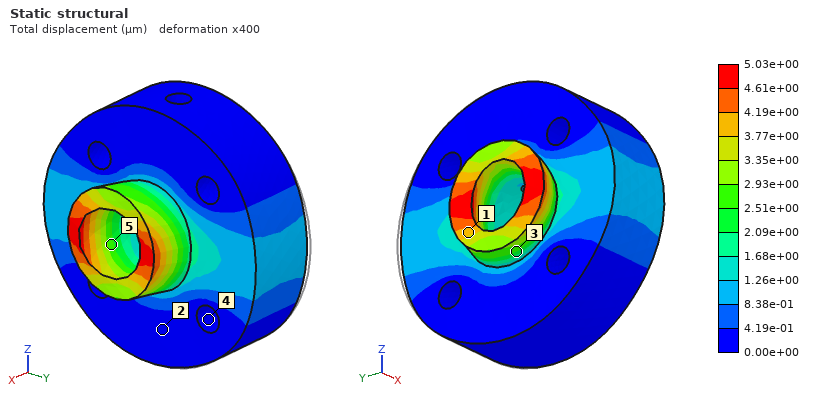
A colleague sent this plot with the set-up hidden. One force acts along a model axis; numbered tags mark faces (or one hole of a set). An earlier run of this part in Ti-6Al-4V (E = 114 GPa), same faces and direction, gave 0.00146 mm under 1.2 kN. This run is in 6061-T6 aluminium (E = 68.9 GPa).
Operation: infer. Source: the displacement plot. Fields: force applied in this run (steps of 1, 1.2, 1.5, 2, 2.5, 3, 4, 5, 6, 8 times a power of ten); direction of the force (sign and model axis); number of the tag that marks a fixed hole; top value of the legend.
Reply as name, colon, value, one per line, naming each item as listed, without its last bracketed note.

force applied in this run: 2.5 kN
direction of the force: -Y
number of the tag that marks a fixed hole: 4
top value of the legend: 5.03e+00 µm
